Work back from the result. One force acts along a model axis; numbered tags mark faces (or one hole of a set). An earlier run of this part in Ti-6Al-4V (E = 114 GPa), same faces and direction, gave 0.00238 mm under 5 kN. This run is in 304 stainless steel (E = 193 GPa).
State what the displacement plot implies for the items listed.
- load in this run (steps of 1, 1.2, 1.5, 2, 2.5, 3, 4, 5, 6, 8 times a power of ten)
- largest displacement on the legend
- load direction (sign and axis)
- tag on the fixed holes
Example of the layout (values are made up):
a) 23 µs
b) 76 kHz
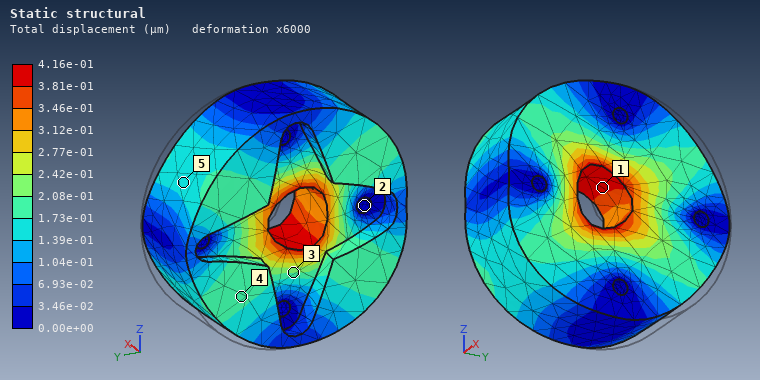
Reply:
a) 1.5 kN
b) 4.16e-01 µm
c) -Y
d) 2
